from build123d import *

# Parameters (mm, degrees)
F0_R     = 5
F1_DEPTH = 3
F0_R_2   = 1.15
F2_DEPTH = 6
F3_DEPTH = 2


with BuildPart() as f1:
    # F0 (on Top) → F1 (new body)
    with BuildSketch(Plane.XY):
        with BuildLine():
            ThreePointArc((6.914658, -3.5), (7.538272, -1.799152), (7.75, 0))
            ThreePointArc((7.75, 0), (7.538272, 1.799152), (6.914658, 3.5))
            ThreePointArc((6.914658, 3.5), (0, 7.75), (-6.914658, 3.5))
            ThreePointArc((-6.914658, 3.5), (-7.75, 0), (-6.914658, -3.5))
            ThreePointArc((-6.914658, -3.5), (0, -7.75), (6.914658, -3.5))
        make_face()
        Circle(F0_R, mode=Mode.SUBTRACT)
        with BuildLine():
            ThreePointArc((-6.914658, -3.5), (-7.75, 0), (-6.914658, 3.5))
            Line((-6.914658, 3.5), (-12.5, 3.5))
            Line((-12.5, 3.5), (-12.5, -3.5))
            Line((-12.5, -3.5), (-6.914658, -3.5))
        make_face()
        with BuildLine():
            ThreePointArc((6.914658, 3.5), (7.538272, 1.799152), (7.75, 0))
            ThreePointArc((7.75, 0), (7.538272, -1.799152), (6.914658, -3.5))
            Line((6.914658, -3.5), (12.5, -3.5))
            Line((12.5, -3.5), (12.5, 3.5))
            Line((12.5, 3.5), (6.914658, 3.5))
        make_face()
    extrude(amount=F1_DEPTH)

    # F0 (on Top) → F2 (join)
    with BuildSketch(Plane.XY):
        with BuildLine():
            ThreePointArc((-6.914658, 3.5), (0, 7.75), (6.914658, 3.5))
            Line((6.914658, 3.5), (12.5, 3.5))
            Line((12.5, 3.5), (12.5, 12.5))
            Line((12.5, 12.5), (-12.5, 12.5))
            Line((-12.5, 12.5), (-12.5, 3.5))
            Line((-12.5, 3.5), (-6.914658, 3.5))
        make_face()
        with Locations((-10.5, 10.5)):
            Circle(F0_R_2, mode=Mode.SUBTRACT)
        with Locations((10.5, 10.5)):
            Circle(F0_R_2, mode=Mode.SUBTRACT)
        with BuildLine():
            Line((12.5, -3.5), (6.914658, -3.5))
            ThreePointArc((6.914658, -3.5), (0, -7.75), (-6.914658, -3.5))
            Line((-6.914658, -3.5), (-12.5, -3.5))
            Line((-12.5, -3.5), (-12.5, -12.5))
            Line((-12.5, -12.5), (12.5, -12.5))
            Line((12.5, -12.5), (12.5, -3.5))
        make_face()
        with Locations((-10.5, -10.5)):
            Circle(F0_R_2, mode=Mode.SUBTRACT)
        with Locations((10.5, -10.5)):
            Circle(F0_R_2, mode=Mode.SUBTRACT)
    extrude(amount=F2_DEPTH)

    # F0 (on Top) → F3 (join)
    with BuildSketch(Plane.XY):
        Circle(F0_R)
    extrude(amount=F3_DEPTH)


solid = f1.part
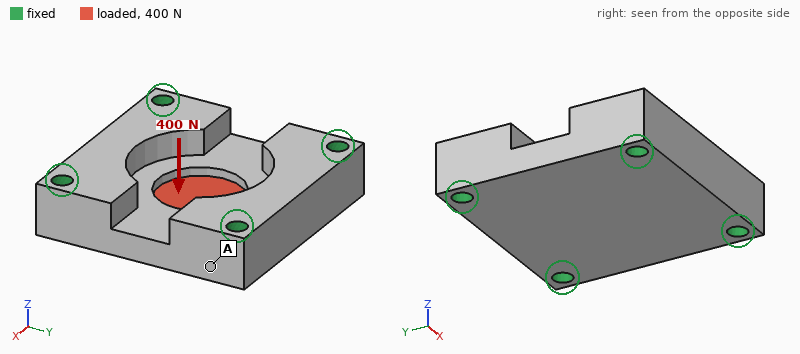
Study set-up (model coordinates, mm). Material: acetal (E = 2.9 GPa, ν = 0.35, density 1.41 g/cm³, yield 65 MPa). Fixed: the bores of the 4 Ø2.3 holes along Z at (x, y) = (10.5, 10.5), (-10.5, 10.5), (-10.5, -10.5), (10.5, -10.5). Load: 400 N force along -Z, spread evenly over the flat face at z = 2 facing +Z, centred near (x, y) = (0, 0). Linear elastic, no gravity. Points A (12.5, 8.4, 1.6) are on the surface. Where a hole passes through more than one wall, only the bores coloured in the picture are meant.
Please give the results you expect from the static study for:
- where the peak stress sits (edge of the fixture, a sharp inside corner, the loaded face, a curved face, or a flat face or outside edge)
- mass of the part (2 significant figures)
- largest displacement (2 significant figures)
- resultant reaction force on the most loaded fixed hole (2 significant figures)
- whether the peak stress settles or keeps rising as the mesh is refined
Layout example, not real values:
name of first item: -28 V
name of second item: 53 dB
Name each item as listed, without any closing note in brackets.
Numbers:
where the peak stress sits: edge of the fixture
mass of the part: 3.9 g
largest displacement: 0.18 mm
resultant reaction force on the most loaded fixed hole: 150 N
whether the peak stress settles or keeps rising as the mesh is refined: keeps rising
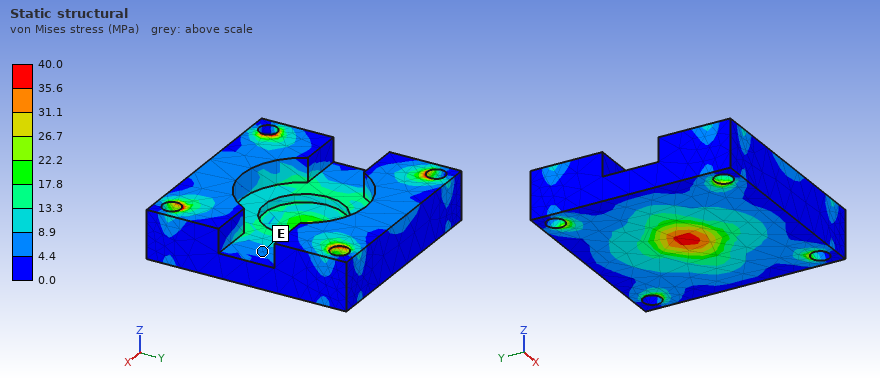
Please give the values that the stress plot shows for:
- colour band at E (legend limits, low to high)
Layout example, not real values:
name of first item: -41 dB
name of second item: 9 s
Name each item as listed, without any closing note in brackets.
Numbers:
colour band at E: 4.4 to 8.9 MPa
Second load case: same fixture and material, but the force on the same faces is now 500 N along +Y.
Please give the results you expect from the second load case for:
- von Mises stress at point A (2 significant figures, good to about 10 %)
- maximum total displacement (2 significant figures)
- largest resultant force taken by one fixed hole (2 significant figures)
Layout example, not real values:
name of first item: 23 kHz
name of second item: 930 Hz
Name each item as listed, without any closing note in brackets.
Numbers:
von Mises stress at point A: 2.4 MPa
maximum total displacement: 51 µm
largest resultant force taken by one fixed hole: 140 N
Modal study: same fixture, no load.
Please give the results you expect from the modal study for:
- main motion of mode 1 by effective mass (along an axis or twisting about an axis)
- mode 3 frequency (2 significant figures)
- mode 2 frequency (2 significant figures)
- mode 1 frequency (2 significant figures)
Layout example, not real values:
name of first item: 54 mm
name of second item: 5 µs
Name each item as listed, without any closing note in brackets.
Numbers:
main motion of mode 1 by effective mass: along Z
mode 3 frequency: 15 kHz
mode 2 frequency: 14 kHz
mode 1 frequency: 11 kHz
